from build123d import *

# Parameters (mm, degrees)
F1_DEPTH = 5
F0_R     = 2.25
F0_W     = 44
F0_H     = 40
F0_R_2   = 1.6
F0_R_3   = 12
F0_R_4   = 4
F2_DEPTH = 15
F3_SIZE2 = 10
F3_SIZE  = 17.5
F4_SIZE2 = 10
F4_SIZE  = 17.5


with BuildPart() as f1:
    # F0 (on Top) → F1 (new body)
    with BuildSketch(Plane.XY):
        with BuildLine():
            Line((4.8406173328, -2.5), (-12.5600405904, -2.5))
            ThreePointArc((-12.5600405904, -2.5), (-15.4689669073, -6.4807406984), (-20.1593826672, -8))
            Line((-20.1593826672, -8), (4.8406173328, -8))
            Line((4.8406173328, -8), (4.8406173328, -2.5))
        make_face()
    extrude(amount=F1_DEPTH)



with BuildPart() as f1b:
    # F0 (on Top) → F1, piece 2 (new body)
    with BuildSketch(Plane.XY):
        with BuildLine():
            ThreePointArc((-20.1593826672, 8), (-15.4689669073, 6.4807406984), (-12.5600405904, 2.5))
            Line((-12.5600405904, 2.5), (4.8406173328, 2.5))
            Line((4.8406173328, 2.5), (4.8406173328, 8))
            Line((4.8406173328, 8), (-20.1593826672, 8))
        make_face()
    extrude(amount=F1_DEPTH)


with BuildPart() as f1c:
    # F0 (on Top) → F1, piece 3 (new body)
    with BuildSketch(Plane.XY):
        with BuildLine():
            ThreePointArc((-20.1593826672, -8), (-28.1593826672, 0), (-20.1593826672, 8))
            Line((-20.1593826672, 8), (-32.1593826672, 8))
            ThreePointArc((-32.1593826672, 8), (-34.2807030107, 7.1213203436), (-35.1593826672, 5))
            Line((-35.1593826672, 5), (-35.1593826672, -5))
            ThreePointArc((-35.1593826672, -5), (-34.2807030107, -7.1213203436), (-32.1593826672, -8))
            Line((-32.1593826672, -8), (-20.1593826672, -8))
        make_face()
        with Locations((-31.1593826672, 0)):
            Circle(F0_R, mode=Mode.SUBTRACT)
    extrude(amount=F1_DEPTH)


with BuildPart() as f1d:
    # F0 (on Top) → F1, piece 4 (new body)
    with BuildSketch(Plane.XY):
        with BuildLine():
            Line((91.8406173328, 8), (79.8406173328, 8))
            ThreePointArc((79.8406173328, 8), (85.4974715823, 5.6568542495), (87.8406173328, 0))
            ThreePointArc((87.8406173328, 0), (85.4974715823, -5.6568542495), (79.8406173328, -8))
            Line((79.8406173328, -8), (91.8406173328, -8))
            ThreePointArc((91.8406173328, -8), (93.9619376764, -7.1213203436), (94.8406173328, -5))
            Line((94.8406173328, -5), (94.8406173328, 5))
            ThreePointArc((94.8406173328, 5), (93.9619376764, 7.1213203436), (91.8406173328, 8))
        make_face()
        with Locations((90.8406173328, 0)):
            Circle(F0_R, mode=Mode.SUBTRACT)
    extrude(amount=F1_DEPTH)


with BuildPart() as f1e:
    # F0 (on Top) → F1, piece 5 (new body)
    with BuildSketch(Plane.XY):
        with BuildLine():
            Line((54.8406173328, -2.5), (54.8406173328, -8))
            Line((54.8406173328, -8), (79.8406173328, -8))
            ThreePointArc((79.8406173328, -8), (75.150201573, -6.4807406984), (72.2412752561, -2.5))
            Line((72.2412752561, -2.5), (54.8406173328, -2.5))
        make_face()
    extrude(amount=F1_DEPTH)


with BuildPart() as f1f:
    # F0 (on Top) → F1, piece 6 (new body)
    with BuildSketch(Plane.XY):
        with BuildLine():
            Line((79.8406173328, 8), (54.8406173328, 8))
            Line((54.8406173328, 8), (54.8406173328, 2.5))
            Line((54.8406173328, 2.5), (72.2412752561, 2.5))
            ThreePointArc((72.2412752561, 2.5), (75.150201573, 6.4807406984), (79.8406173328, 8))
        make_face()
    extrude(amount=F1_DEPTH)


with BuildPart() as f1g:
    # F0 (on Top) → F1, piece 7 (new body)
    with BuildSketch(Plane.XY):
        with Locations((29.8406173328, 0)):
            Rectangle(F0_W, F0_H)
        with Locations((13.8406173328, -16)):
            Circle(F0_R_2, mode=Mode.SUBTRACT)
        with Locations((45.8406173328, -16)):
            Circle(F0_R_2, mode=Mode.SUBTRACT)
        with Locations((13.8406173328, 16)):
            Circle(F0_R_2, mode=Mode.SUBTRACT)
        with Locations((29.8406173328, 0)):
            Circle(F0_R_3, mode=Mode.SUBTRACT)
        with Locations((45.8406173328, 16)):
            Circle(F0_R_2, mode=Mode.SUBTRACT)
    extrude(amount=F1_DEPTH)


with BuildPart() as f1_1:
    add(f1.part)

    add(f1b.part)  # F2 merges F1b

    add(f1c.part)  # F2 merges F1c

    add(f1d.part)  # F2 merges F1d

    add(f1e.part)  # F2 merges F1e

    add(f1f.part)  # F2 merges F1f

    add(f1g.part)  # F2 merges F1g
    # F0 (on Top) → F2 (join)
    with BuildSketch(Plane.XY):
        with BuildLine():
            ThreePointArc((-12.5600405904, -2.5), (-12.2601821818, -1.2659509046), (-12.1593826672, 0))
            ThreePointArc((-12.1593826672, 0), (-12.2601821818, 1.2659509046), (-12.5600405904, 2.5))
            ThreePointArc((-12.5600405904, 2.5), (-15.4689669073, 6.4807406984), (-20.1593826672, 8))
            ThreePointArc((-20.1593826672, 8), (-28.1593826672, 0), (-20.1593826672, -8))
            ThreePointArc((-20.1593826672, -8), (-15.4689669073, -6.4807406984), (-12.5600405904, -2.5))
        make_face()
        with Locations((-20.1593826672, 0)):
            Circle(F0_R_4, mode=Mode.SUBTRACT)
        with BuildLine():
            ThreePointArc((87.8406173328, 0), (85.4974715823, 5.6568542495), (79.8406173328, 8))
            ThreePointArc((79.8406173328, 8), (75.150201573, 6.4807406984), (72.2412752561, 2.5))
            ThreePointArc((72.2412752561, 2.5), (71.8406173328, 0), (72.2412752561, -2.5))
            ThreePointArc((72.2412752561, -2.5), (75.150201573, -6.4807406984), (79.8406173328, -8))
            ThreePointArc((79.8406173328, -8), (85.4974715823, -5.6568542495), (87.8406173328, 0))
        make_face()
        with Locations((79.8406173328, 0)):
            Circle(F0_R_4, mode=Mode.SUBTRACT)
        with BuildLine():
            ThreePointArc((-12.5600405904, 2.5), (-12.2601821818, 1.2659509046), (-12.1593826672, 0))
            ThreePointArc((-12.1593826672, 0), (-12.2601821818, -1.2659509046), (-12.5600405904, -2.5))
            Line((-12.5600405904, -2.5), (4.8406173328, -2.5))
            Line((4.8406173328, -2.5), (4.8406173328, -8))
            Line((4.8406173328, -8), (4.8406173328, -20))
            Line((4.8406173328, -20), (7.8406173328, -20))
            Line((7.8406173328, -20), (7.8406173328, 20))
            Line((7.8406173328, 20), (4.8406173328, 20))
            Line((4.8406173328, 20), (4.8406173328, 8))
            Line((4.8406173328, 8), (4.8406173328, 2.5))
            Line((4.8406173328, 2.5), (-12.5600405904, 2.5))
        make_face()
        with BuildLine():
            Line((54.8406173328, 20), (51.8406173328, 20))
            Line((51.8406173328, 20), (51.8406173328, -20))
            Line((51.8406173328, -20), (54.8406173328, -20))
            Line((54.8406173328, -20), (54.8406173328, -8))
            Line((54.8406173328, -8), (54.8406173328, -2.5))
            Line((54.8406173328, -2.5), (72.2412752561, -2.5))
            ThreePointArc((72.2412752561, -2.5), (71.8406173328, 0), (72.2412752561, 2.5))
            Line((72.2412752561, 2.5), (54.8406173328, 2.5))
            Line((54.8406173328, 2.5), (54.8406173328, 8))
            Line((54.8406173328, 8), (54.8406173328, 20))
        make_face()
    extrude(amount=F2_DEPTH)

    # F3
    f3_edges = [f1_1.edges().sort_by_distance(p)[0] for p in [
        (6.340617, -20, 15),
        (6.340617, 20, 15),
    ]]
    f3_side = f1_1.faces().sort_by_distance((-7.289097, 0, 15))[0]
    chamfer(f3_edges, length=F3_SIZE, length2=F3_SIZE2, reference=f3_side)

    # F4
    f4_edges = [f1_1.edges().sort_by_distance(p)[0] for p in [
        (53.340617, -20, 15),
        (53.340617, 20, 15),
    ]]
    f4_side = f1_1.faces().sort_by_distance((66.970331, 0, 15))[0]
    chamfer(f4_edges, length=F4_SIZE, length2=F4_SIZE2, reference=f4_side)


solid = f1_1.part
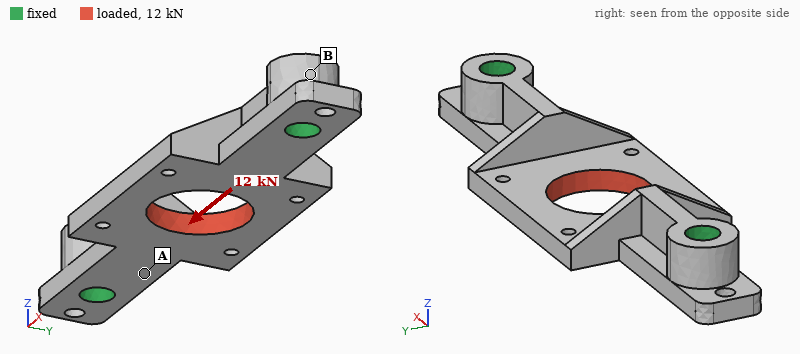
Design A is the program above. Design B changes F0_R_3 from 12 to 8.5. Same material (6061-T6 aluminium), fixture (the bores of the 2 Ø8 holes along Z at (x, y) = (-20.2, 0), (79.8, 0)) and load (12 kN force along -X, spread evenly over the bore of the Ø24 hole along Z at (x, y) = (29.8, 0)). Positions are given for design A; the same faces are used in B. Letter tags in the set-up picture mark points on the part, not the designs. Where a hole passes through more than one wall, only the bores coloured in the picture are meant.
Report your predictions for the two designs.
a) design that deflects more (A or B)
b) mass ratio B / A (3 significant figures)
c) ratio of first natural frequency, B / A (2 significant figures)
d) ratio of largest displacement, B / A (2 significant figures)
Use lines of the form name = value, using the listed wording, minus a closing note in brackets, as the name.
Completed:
design that deflects more = A
mass ratio B / A = 1.06
ratio of first natural frequency, B / A = 0.98
ratio of largest displacement, B / A = 0.90
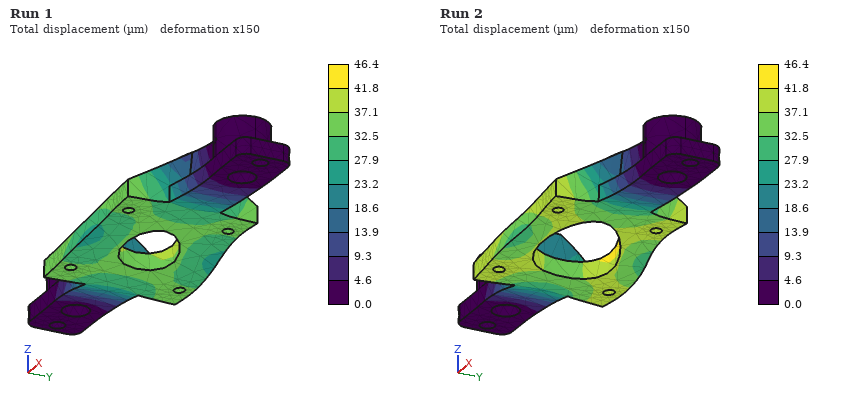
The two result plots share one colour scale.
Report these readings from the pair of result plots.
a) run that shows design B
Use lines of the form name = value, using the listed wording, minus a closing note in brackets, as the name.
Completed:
run that shows design B = Run 1
